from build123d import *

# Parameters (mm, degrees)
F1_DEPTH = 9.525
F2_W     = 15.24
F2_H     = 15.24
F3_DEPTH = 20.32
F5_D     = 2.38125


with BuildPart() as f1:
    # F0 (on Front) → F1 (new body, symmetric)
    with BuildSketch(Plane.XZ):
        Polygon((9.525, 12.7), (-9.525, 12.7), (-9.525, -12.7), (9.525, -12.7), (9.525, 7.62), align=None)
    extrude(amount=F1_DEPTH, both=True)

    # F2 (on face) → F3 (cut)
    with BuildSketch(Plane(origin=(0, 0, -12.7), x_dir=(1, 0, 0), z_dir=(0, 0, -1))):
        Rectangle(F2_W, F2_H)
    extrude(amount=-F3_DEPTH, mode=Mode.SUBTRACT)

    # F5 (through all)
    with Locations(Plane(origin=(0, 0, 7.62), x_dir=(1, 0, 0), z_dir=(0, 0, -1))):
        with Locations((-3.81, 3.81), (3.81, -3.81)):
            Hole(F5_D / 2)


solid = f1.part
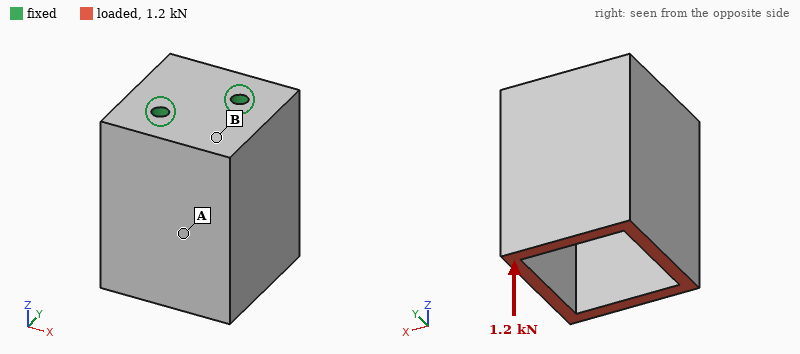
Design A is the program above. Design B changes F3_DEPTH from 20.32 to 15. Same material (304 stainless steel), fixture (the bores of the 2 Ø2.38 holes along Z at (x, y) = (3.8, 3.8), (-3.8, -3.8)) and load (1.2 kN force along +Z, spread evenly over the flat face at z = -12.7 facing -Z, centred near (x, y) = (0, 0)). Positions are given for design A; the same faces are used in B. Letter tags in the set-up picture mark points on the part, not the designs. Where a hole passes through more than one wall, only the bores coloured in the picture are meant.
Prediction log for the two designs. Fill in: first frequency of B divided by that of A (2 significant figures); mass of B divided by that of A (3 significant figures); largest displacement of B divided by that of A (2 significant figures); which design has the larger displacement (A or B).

2.1
1.27
0.46
A
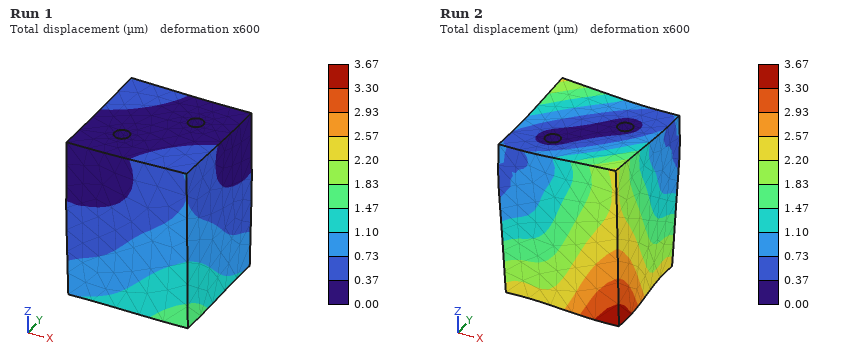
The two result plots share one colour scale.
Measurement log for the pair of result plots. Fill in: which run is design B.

Run 1
